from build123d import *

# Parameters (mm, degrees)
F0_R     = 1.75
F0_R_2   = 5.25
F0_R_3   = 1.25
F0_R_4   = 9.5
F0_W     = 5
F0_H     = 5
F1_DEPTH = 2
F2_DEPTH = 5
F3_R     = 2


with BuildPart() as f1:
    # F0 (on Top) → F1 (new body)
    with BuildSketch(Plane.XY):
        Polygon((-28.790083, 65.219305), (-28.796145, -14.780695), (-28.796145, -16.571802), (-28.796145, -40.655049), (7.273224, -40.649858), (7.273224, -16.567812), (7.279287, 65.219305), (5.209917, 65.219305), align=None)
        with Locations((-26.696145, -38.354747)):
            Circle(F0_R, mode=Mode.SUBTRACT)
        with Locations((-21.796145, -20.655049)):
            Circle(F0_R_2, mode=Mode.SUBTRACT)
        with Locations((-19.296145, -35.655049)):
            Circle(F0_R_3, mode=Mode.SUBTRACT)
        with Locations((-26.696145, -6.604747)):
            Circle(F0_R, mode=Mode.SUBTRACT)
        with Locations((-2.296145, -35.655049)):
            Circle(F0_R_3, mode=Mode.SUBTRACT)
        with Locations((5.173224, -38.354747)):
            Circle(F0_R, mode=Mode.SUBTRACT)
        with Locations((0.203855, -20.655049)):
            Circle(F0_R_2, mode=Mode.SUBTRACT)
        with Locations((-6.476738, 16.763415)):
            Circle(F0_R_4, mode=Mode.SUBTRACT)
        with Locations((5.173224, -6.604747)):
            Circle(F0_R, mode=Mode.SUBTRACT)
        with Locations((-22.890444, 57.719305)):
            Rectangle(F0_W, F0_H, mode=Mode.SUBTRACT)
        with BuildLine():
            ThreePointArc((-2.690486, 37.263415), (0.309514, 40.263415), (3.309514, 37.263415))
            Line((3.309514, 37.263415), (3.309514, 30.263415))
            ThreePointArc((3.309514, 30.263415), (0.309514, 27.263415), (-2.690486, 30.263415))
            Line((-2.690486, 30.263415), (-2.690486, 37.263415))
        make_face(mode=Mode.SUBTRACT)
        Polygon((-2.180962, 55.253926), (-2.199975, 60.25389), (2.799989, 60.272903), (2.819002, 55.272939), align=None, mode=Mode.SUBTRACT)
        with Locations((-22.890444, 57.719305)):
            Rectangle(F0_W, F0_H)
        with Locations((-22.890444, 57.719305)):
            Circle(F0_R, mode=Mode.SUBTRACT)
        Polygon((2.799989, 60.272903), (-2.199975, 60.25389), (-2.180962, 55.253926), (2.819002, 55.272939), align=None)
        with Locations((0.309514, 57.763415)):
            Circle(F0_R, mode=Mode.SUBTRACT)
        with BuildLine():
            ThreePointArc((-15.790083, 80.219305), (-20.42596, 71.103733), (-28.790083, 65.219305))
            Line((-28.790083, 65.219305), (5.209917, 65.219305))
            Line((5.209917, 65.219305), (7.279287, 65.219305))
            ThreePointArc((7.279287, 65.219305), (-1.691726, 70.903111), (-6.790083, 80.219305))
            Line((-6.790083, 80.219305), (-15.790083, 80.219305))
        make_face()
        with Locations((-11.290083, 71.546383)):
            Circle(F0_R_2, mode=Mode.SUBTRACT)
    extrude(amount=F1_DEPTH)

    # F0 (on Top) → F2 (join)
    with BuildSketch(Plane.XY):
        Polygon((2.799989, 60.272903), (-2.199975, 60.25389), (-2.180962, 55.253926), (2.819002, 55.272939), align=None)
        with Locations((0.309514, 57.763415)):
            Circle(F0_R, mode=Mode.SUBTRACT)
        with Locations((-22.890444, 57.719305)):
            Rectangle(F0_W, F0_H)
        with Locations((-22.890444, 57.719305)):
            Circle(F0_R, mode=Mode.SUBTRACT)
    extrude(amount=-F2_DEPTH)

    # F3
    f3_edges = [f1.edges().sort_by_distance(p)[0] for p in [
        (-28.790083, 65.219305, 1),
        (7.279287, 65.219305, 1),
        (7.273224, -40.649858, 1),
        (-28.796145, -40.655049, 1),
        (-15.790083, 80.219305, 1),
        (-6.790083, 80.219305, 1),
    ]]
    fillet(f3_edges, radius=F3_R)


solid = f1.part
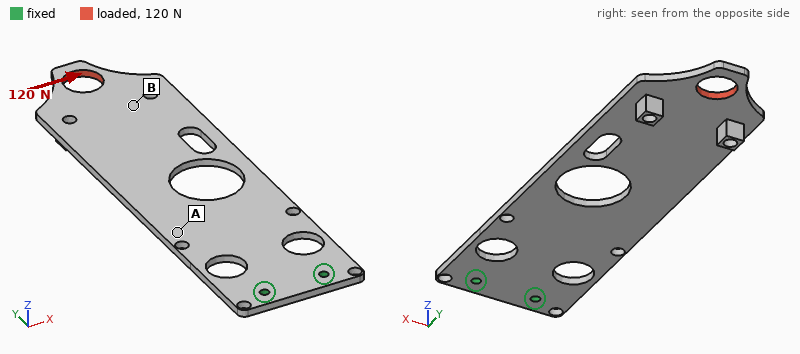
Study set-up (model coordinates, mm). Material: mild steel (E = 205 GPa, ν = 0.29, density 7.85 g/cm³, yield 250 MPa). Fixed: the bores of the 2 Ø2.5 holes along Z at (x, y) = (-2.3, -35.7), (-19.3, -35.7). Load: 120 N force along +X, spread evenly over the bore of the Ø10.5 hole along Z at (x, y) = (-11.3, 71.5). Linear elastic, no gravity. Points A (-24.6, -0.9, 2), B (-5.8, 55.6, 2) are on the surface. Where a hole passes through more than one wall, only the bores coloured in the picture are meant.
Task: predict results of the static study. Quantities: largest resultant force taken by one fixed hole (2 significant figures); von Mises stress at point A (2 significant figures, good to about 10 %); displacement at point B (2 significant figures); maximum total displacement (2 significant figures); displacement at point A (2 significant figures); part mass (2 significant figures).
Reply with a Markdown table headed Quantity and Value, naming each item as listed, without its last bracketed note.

| Quantity | Value |
|---|---|
| largest resultant force taken by one fixed hole | 690 N |
| von Mises stress at point A | 16 MPa |
| displacement at point B | 65 µm |
| maximum total displacement | 89 µm |
| displacement at point A | 18 µm |
| part mass | 55 g |
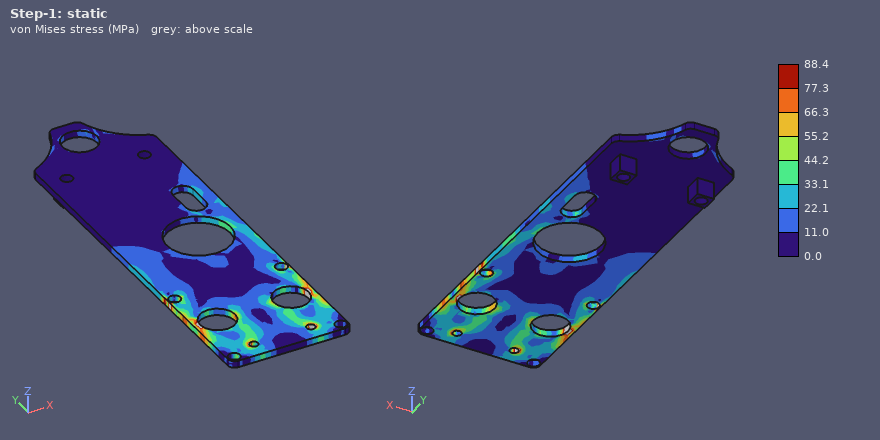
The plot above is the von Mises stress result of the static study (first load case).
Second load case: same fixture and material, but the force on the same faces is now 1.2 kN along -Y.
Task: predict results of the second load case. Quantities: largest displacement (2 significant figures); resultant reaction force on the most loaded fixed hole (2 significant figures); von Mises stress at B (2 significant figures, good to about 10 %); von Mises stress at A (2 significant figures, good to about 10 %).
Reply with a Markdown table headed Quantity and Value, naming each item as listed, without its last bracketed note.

| Quantity | Value |
|---|---|
| largest displacement | 20 µm |
| resultant reaction force on the most loaded fixed hole | 630 N |
| von Mises stress at B | 20 MPa |
| von Mises stress at A | 21 MPa |
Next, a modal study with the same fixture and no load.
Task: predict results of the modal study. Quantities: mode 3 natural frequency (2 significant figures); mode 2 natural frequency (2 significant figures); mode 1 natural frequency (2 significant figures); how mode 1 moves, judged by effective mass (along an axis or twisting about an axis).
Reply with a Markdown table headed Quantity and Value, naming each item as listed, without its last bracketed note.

| Quantity | Value |
|---|---|
| mode 3 natural frequency | 820 Hz |
| mode 2 natural frequency | 780 Hz |
| mode 1 natural frequency | 120 Hz |
| how mode 1 moves, judged by effective mass | along Z |
